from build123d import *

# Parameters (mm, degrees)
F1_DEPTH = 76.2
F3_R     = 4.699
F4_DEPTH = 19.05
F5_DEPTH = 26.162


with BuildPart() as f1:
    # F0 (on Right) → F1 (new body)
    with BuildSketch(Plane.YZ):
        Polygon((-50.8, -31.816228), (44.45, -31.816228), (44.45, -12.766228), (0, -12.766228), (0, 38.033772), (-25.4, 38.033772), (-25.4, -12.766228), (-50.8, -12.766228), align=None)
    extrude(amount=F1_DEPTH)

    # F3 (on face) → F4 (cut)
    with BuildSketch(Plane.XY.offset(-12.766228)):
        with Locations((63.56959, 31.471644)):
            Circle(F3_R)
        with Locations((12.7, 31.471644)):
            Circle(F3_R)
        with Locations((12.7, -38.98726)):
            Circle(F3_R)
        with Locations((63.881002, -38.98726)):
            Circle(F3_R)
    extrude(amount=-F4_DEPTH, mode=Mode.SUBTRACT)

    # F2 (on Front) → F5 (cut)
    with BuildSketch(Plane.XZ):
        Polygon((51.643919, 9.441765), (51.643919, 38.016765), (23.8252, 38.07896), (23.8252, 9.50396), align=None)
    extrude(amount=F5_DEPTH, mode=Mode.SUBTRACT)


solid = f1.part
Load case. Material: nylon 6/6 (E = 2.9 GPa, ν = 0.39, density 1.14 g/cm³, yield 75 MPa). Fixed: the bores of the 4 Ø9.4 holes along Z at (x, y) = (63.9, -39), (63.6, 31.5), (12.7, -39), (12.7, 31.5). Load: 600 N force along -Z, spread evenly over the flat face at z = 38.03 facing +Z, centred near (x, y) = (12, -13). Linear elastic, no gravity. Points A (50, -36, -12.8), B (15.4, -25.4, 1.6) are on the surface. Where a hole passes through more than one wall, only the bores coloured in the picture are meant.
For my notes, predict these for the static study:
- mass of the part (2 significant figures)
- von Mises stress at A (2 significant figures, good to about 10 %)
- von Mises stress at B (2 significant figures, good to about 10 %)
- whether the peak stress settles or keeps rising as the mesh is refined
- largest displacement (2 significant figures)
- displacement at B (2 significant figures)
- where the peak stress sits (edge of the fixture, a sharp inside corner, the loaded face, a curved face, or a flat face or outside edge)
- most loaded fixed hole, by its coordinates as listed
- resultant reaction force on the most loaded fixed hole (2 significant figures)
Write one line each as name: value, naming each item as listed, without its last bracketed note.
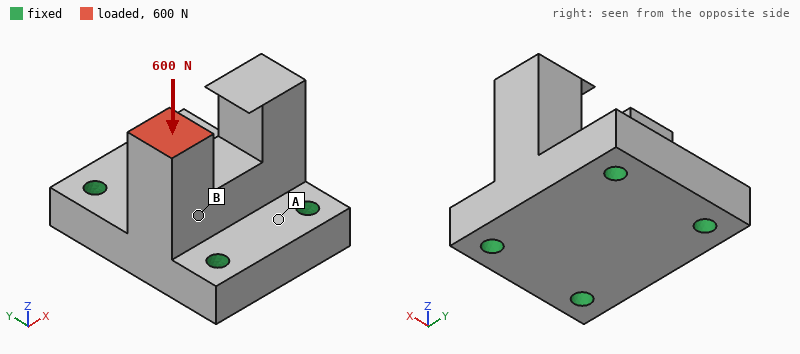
mass of the part: 240 g
von Mises stress at A: 0.33 MPa
von Mises stress at B: 0.91 MPa
whether the peak stress settles or keeps rising as the mesh is refined: keeps rising
largest displacement: 60 µm
displacement at B: 23 µm
where the peak stress sits: edge of the fixture
most loaded fixed hole, by its coordinates as listed: (12.7, -39)
resultant reaction force on the most loaded fixed hole: 390 N
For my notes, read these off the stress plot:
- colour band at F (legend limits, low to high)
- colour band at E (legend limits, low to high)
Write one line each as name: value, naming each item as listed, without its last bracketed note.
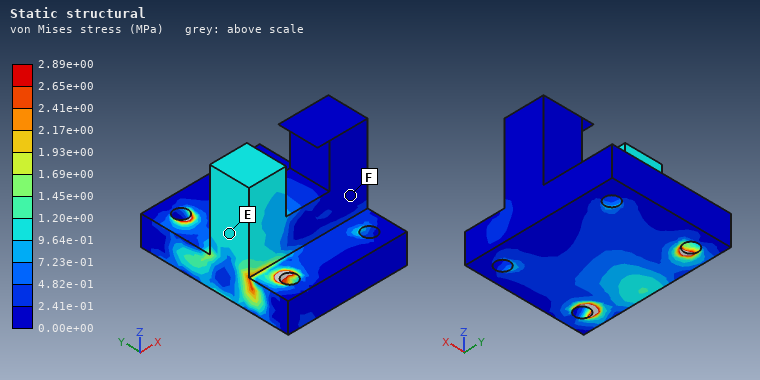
colour band at F: 0.00e+00 to 2.41e-01 MPa
colour band at E: 9.64e-01 to 1.20e+00 MPa
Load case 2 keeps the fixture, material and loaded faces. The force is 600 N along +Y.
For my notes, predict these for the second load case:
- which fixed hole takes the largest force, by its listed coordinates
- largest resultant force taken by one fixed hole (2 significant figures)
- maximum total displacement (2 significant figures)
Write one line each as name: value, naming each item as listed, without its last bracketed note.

which fixed hole takes the largest force, by its listed coordinates: (12.7, -39)
largest resultant force taken by one fixed hole: 530 N
maximum total displacement: 0.41 mm
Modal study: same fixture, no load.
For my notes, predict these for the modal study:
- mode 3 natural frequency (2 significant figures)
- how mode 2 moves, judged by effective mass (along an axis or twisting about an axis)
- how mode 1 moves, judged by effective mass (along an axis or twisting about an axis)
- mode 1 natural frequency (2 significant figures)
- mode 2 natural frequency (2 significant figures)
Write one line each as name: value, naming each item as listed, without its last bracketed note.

mode 3 natural frequency: 2100 Hz
how mode 2 moves, judged by effective mass: along X
how mode 1 moves, judged by effective mass: along Y
mode 1 natural frequency: 1800 Hz
mode 2 natural frequency: 1900 Hz
